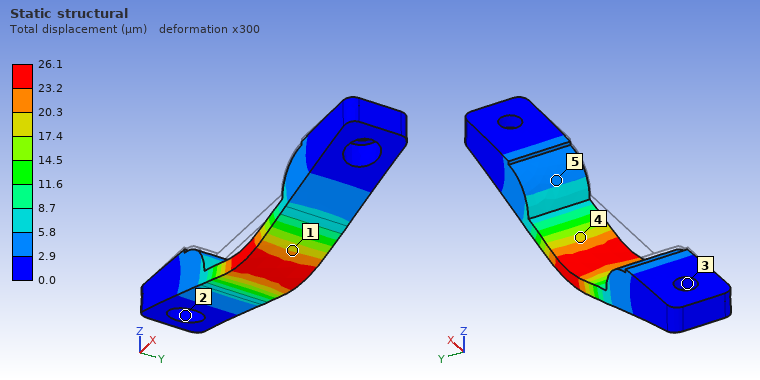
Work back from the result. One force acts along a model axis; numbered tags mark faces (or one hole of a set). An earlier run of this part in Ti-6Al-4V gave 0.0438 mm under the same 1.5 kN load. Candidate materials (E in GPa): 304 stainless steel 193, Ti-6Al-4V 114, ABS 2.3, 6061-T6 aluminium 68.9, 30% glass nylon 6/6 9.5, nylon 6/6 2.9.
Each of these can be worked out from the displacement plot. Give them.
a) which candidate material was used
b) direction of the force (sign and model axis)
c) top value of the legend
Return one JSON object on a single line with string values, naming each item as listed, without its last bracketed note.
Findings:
{"which candidate material was used": "304 stainless steel", "direction of the force": "-Z", "top value of the legend": "26.1 µm"}
